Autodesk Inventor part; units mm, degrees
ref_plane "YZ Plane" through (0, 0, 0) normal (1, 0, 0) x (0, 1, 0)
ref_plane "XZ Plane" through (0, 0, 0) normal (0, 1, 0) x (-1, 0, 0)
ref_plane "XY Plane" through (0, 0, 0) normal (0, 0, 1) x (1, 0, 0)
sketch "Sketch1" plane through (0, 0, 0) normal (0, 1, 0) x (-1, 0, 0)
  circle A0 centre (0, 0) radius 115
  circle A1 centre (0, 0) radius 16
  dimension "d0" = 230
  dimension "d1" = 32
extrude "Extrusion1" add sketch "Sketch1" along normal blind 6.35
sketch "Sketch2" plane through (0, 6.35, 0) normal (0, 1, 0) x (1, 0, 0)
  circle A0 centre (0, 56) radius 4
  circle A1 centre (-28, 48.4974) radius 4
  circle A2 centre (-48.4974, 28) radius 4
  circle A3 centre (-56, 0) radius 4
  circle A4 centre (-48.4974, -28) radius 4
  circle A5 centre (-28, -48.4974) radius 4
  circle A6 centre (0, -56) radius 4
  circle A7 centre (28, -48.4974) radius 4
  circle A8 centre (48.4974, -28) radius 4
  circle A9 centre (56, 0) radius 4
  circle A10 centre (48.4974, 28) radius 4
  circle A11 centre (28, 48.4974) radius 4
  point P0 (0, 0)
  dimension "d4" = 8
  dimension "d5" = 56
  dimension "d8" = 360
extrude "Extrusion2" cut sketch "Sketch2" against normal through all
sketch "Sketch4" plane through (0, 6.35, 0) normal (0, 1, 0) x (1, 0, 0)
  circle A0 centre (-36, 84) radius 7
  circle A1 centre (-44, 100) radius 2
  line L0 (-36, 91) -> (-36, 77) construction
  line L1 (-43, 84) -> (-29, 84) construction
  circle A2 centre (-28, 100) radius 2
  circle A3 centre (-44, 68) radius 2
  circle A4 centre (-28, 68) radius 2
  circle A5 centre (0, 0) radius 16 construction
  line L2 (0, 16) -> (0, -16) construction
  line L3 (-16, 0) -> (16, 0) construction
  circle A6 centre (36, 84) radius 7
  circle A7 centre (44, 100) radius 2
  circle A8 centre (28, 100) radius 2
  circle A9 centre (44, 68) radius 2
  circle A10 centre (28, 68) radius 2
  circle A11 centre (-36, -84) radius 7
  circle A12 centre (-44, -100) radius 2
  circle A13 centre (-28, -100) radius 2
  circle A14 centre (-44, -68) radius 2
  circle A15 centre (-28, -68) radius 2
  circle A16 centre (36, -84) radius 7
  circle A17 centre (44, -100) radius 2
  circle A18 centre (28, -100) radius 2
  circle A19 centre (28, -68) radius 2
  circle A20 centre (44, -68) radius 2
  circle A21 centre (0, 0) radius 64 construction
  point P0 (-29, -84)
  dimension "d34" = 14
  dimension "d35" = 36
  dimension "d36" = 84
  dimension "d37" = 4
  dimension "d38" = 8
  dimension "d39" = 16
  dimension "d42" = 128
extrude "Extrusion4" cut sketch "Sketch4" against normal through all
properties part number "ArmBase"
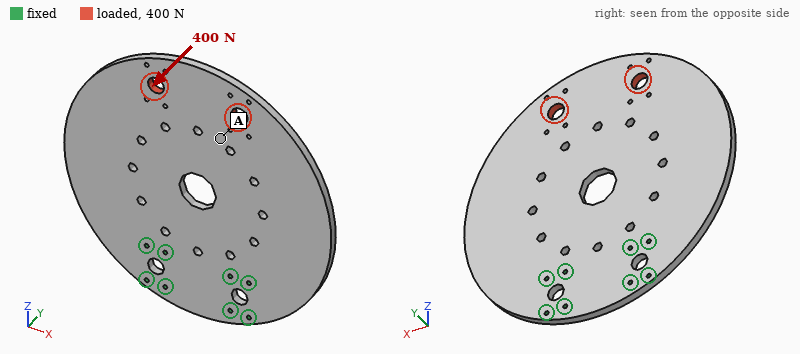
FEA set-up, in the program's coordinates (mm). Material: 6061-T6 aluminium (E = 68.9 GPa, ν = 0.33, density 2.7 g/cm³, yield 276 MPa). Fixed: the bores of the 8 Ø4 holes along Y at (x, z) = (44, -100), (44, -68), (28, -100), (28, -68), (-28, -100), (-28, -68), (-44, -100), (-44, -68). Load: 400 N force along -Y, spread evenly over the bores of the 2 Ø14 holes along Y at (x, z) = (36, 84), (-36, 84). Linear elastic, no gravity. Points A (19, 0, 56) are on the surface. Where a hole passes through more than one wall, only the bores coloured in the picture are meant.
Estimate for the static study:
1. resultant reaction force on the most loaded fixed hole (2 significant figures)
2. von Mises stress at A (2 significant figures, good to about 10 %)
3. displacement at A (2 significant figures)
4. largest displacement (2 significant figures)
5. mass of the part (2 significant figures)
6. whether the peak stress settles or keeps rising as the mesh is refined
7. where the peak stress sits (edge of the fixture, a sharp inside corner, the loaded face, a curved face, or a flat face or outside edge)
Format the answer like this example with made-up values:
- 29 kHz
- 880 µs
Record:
- 340 N
- 8.7 MPa
- 1.4 mm
- 2.4 mm
- 670 g
- keeps rising
- edge of the fixture
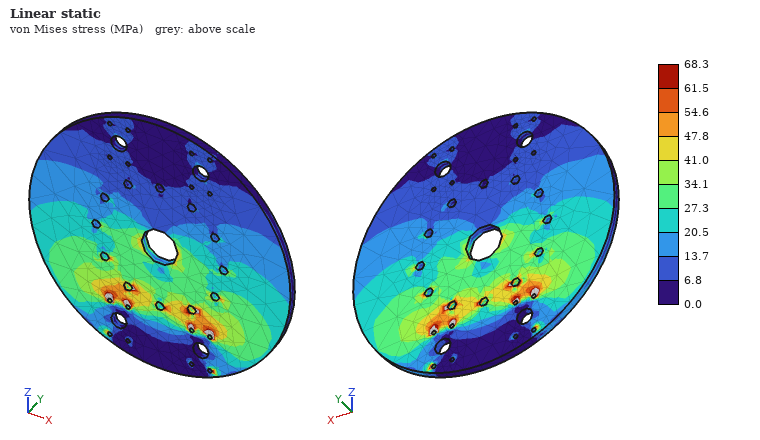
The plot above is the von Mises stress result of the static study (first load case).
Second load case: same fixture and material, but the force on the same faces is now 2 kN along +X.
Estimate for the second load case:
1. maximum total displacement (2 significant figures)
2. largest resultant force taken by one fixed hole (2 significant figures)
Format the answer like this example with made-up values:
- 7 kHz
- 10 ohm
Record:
- 51 µm
- 1.9 kN
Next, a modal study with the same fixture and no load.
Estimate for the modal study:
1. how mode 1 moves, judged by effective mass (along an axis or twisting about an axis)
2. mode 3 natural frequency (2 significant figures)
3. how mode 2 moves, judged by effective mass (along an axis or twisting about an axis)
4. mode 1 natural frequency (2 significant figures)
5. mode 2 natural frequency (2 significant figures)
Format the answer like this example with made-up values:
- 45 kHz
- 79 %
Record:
- along Y
- 720 Hz
- twisting about Z
- 170 Hz
- 350 Hz
